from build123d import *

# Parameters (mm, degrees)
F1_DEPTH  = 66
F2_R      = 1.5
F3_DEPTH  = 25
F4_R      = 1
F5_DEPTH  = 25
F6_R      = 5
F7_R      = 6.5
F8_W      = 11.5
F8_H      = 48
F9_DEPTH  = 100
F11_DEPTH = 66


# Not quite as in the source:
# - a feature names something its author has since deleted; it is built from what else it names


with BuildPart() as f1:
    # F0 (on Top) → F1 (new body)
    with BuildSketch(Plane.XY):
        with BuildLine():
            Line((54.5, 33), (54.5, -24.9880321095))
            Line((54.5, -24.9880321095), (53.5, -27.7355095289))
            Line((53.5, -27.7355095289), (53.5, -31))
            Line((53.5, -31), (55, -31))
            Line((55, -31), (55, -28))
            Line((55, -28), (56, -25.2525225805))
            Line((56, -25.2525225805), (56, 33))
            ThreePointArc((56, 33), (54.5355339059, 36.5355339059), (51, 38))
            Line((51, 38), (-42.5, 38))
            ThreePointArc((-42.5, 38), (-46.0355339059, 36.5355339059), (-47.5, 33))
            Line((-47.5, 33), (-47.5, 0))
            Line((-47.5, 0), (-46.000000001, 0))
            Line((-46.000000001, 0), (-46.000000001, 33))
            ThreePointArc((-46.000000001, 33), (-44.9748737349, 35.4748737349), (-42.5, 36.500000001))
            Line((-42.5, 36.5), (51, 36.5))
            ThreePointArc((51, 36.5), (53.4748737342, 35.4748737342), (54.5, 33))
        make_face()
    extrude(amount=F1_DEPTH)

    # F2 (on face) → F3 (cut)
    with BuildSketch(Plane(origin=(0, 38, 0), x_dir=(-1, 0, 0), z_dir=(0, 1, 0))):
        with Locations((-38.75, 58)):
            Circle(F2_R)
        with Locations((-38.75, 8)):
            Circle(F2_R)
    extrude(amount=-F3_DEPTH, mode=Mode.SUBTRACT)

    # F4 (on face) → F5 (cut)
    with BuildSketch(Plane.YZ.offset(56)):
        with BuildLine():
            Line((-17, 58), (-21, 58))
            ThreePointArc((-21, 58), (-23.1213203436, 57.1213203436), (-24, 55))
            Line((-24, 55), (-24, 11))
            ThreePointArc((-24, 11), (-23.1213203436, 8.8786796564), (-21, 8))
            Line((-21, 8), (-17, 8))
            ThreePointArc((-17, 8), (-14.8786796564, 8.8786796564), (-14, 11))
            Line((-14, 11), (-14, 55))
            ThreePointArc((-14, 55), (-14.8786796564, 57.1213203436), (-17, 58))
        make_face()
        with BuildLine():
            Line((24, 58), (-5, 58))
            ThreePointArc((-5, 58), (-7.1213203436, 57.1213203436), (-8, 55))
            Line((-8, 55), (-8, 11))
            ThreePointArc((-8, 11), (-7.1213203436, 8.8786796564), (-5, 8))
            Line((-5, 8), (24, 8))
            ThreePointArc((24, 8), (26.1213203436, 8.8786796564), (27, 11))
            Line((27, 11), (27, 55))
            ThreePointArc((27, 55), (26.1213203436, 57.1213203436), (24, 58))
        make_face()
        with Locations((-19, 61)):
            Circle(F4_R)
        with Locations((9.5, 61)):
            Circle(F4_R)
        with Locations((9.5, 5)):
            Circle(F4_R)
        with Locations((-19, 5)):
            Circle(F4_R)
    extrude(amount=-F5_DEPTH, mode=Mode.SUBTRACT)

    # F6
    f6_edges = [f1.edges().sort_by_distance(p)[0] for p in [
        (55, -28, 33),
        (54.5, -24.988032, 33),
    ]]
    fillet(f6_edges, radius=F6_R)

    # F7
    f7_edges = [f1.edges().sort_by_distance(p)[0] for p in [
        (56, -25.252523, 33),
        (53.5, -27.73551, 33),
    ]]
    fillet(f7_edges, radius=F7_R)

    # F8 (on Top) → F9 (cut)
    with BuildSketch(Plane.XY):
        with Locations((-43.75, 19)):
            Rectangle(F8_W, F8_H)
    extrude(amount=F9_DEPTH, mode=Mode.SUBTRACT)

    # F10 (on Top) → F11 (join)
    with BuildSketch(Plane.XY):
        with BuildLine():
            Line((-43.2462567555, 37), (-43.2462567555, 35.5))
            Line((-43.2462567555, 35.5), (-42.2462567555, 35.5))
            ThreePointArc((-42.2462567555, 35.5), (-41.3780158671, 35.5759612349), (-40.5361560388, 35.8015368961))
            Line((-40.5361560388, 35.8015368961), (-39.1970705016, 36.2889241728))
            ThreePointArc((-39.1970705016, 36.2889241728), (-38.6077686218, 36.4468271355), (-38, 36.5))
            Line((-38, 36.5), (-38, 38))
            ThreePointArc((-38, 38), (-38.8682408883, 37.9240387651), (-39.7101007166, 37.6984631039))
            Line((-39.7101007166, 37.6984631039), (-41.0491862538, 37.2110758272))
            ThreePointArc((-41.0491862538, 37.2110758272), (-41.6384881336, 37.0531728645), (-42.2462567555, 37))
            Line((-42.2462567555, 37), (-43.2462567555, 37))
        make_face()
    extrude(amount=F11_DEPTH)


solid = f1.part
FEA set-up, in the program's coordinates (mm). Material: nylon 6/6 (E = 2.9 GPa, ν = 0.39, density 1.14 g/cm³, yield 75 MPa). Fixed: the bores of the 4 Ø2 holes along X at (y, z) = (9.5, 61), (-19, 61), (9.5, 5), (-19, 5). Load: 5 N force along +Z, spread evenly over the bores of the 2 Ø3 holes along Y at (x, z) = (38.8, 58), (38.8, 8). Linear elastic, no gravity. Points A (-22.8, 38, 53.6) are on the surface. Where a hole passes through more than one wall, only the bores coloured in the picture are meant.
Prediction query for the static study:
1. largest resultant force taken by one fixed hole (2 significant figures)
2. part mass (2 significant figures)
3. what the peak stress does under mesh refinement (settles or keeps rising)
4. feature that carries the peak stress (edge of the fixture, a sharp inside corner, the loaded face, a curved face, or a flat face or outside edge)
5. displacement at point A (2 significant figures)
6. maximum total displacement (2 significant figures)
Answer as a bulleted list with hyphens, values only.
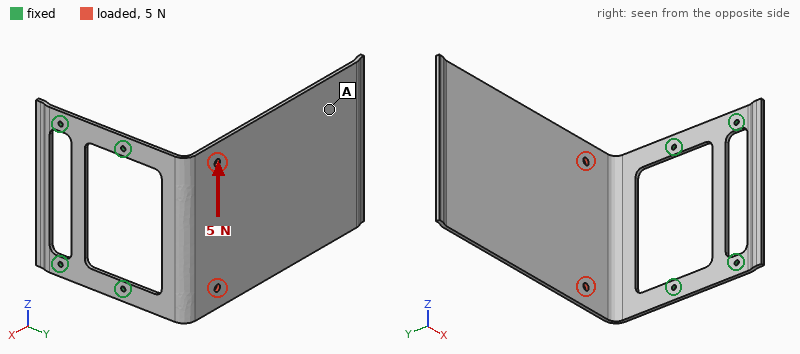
- 3.4 N
- 15 g
- keeps rising
- edge of the fixture
- 1.2 mm
- 1.6 mm
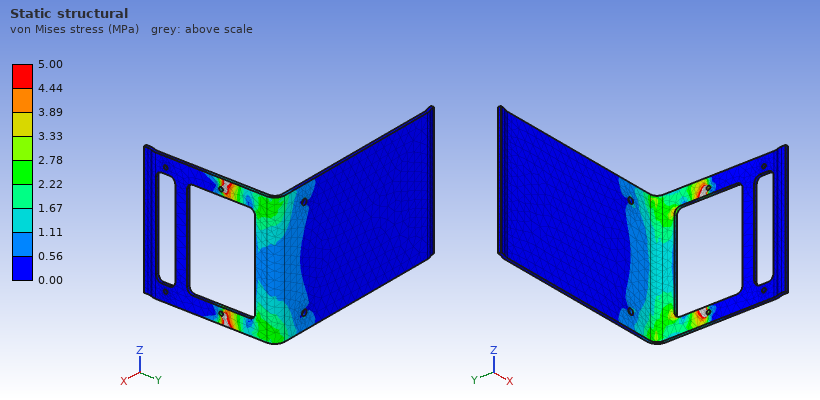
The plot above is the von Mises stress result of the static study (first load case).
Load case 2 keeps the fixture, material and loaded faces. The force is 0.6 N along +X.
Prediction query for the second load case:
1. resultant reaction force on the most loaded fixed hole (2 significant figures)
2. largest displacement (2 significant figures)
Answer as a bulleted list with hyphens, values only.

- 0.31 N
- 1.6 mm
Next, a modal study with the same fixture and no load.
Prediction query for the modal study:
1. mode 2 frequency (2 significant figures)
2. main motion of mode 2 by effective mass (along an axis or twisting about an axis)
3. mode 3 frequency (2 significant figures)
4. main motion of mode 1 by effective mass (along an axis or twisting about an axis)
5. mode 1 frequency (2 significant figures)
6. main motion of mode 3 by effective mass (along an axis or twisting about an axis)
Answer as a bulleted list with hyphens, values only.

- 58 Hz
- along Z
- 110 Hz
- along Y
- 18 Hz
- along X
